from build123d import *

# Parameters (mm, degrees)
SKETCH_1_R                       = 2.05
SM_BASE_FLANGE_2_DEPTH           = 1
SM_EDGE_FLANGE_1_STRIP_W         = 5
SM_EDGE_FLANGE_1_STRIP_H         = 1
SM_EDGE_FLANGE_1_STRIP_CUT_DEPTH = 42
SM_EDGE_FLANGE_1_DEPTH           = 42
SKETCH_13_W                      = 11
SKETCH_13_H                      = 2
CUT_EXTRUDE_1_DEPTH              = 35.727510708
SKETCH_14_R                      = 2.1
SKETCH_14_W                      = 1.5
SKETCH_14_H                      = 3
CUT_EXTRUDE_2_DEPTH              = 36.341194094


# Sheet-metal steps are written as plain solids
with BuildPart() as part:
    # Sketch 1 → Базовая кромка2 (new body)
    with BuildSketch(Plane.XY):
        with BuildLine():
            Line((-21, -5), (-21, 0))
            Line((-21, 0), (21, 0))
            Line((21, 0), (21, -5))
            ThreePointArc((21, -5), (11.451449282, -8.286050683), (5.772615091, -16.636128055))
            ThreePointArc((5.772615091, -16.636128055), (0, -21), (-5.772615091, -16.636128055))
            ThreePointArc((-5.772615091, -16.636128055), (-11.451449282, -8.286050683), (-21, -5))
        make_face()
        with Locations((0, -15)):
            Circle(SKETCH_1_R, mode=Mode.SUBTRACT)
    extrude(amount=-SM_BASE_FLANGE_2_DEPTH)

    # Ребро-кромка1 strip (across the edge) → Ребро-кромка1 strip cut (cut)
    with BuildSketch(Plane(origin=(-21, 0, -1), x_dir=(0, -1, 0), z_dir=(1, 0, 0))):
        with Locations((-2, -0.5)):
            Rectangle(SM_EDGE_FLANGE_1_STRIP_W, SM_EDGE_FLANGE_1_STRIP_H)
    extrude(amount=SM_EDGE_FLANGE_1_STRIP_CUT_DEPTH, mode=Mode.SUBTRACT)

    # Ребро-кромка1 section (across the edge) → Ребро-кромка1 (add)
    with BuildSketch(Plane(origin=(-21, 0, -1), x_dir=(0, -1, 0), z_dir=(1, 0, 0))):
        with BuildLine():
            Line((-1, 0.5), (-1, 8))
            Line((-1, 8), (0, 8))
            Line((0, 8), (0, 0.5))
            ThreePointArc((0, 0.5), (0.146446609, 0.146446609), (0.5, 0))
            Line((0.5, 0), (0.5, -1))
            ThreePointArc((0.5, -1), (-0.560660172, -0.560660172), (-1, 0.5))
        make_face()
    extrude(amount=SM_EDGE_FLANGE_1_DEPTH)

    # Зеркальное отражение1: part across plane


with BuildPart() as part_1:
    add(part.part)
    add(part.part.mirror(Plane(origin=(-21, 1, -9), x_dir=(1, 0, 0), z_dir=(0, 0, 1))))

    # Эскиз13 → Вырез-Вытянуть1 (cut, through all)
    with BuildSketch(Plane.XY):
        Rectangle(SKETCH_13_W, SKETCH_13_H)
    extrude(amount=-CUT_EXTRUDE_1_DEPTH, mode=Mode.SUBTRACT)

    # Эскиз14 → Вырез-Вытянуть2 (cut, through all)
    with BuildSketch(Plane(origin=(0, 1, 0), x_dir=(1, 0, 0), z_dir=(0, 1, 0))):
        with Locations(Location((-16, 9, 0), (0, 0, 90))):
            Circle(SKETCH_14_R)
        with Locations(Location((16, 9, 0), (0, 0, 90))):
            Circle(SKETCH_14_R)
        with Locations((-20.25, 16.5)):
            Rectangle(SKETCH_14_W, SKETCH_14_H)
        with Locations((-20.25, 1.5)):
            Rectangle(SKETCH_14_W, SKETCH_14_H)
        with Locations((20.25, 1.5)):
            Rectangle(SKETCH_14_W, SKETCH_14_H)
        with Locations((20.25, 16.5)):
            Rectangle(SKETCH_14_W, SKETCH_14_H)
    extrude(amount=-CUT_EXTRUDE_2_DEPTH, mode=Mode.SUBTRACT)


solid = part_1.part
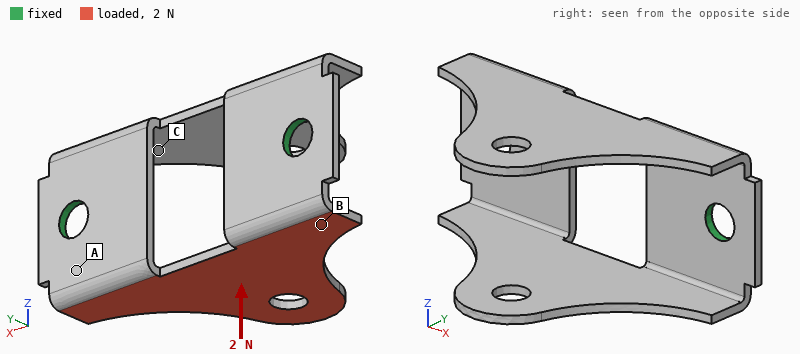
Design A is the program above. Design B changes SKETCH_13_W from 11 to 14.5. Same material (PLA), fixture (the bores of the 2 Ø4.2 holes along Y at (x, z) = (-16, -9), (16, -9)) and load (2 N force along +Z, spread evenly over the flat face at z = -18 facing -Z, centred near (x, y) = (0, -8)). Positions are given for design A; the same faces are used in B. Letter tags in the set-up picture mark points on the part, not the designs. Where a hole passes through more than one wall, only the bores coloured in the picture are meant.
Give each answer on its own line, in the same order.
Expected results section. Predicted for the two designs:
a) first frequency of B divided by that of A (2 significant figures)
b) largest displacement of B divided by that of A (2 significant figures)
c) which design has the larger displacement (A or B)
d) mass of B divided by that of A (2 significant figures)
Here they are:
0.94
1.1
B
0.95
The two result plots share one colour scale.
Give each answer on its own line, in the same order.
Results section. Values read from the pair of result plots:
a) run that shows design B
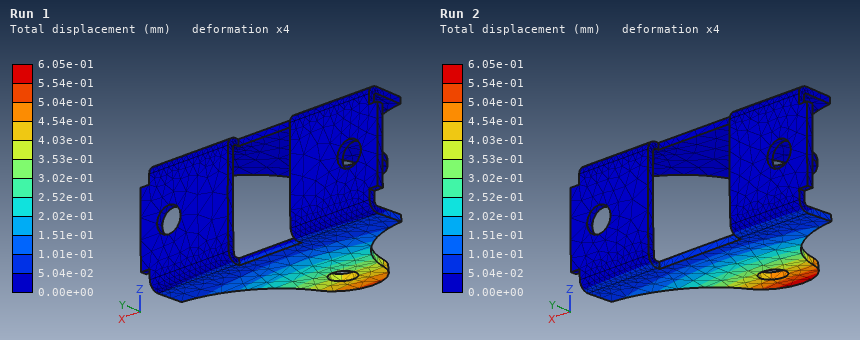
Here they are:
Run 2
